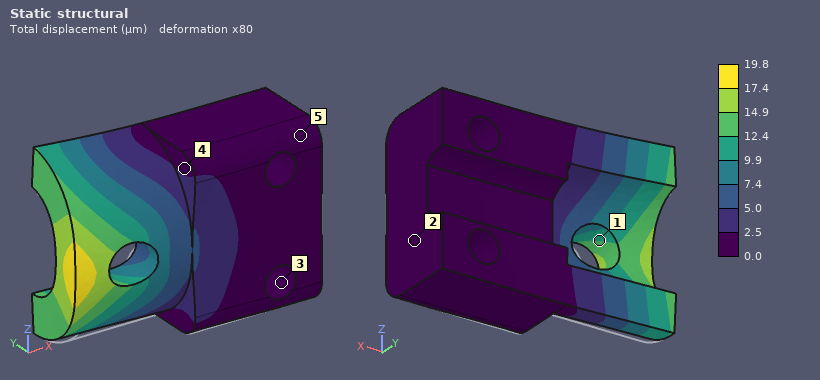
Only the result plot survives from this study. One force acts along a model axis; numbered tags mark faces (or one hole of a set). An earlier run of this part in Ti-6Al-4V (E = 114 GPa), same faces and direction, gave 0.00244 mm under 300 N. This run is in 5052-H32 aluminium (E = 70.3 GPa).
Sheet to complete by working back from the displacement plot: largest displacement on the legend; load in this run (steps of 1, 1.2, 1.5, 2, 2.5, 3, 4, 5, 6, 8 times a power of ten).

19.8 µm
1.5 kN
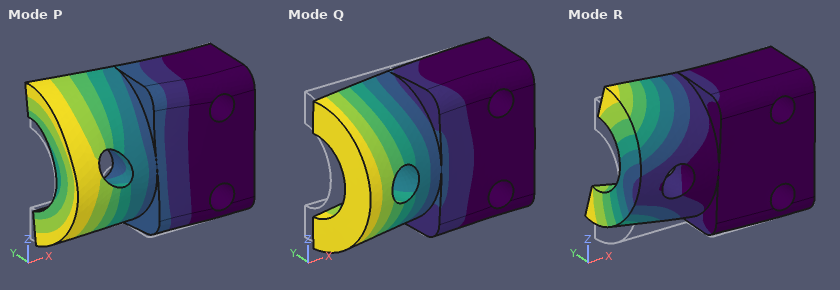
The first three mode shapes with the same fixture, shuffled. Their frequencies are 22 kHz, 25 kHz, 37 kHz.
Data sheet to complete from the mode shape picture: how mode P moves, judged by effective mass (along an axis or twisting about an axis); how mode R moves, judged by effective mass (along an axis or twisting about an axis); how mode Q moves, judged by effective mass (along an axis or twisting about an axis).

along Z
along Z
along Y
